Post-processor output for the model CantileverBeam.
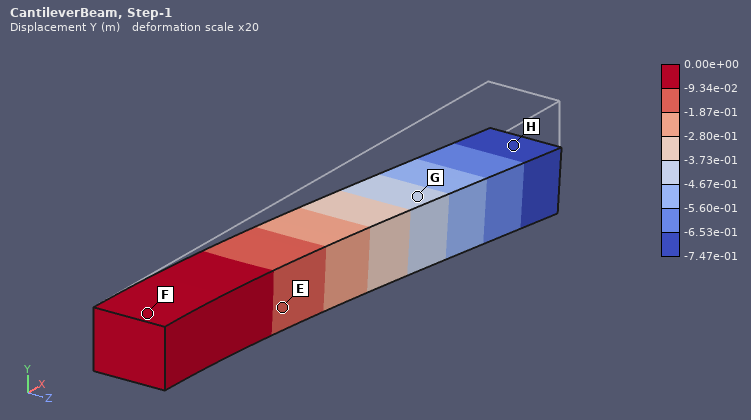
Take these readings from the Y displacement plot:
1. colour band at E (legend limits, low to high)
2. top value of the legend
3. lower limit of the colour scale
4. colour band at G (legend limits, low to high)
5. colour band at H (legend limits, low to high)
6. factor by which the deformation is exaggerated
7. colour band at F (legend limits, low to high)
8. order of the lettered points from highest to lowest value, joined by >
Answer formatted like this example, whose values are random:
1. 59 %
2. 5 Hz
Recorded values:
1. -1.87e-01 to -9.34e-02 m
2. 0.00e+00 m
3. -7.47e-01 m
4. -4.67e-01 to -3.73e-01 m
5. -7.47e-01 to -6.53e-01 m
6. 20
7. -9.34e-02 to 0.00e+00 m
8. F > E > G > H
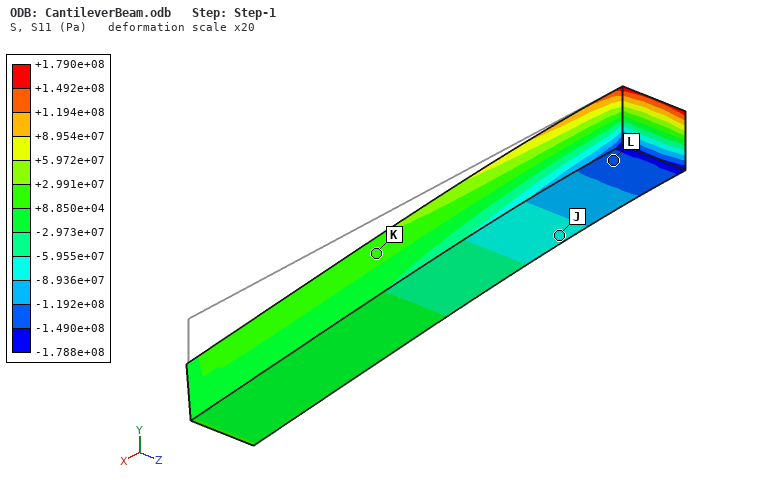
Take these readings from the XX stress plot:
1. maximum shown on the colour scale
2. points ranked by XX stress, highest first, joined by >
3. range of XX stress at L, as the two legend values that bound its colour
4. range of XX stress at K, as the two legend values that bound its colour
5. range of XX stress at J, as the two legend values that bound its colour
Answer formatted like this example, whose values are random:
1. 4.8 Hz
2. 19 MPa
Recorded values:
1. +1.790e+08 Pa
2. K > J > L
3. -1.490e+08 to -1.192e+08 Pa
4. +8.850e+04 to +2.991e+07 Pa
5. -8.936e+07 to -5.955e+07 Pa
